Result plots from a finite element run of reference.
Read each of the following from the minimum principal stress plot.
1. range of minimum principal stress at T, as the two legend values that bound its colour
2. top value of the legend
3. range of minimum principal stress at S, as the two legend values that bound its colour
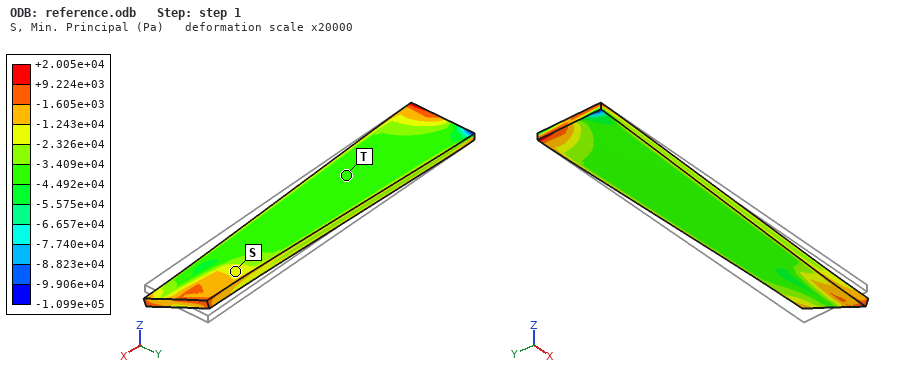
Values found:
-4.492e+04 to -3.409e+04 Pa
+2.005e+04 Pa
-2.326e+04 to -1.243e+04 Pa
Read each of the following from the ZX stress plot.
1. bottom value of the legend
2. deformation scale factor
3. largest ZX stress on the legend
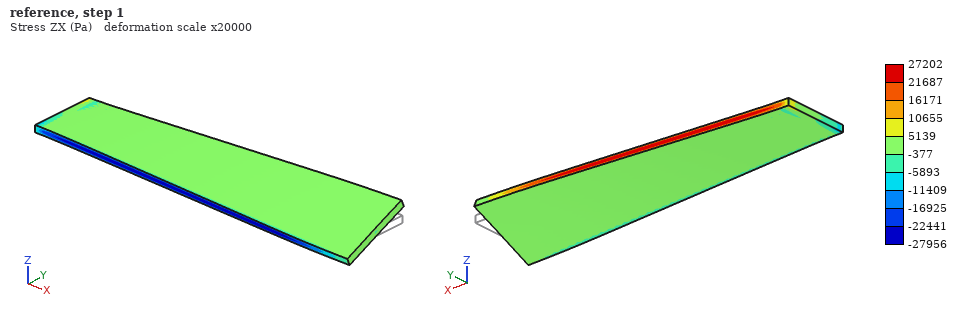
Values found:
-27956 Pa
20000
27202 Pa
